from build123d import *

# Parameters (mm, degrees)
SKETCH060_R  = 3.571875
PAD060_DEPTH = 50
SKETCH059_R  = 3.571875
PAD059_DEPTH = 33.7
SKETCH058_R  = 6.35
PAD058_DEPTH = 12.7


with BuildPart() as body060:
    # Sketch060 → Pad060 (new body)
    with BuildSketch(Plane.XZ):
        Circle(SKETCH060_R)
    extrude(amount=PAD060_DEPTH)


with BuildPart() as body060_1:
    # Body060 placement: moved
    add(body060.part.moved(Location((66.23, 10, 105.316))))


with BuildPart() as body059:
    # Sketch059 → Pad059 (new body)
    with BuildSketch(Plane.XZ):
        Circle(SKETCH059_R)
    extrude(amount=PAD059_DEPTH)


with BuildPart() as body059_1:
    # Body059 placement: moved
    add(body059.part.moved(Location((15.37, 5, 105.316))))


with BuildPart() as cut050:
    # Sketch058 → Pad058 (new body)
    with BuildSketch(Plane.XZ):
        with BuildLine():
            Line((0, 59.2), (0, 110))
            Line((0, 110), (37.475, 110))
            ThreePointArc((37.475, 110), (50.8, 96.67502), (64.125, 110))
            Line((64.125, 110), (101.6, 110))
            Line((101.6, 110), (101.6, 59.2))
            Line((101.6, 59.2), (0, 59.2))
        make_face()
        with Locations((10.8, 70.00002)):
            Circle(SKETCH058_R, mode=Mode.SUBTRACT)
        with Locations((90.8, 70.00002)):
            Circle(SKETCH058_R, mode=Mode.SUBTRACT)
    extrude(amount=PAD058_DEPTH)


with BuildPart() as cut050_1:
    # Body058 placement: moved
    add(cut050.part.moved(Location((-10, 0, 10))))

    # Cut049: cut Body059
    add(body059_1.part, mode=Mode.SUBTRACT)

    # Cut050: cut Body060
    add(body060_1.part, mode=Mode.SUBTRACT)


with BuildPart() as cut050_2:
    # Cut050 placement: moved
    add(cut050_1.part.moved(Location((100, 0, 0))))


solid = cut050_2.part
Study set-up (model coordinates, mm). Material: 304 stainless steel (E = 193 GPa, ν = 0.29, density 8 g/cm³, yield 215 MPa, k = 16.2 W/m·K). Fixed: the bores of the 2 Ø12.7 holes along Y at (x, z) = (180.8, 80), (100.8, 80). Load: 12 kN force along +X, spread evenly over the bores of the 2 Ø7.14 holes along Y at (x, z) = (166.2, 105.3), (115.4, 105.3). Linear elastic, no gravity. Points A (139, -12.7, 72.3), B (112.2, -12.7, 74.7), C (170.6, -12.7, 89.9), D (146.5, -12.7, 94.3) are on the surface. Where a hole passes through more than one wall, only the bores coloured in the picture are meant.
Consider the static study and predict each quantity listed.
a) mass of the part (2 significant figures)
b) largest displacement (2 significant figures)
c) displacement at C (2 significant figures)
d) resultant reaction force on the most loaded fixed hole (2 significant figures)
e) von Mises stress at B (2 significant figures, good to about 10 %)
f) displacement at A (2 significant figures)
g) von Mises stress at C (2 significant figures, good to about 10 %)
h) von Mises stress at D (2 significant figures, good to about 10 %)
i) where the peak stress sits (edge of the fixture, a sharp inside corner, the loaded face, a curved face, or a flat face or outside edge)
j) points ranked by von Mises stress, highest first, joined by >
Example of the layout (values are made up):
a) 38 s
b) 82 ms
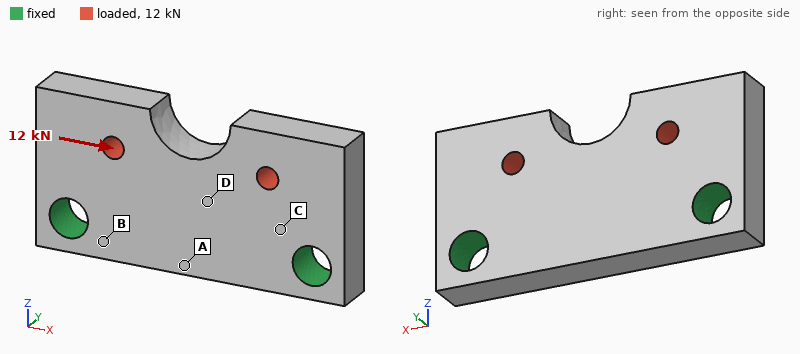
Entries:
a) 460 g
b) 5.6 µm
c) 1.4 µm
d) 6.8 kN
e) 9.3 MPa
f) 1.2 µm
g) 22 MPa
h) 17 MPa
i) edge of the fixture
j) C > D > B > A
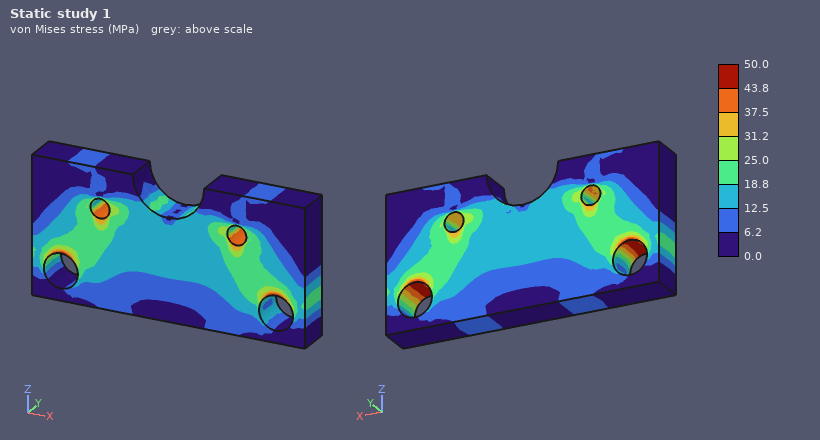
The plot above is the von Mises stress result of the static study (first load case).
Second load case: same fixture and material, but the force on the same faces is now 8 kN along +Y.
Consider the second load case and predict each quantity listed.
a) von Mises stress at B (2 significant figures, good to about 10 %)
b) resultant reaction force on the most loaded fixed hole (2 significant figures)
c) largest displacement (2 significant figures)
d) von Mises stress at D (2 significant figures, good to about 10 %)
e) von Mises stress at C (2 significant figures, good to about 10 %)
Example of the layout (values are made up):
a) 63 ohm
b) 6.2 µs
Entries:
a) 43 MPa
b) 4.0 kN
c) 44 µm
d) 21 MPa
e) 61 MPa
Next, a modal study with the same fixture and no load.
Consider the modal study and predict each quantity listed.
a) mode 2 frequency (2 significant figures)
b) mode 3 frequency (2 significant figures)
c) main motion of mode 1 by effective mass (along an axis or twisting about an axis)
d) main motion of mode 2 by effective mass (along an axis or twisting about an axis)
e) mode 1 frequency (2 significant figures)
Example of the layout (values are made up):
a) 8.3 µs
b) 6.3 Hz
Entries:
a) 7900 Hz
b) 9900 Hz
c) along Y
d) twisting about Z
e) 5600 Hz
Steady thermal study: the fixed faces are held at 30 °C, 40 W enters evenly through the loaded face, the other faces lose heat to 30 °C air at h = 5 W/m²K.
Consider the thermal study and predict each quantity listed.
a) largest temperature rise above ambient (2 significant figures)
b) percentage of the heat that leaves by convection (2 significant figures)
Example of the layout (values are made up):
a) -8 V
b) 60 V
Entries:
a) 79 K
b) 6.0 %
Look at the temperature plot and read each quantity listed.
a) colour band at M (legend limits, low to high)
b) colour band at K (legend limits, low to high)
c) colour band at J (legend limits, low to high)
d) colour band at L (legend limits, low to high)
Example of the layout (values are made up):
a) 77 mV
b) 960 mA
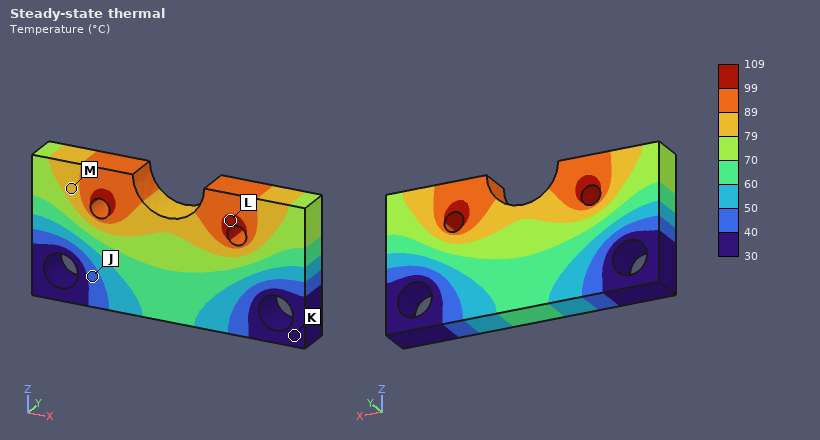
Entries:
a) 79 to 89 °C
b) 30 to 40 °C
c) 40 to 50 °C
d) 99 to 109 °C
